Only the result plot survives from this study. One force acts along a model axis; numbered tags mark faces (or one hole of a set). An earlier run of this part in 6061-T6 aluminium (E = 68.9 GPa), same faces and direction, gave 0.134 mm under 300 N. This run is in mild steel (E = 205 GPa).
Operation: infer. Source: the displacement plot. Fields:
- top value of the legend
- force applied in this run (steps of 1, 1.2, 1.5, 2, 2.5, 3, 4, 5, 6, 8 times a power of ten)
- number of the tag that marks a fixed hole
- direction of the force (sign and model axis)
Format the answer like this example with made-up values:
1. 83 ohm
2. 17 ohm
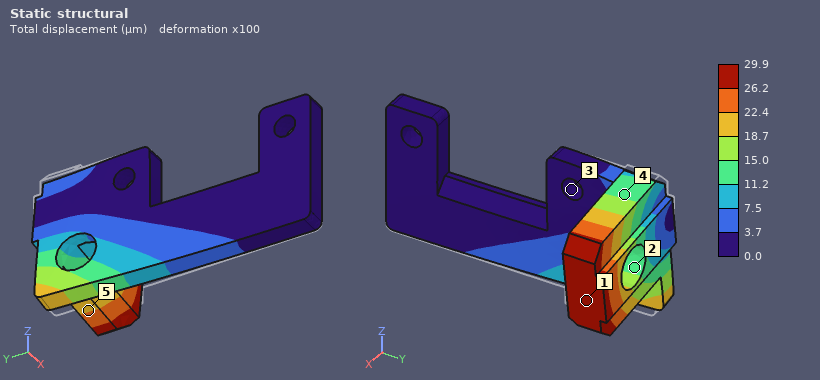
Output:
1. 29.9 µm
2. 200 N
3. 3
4. -Z
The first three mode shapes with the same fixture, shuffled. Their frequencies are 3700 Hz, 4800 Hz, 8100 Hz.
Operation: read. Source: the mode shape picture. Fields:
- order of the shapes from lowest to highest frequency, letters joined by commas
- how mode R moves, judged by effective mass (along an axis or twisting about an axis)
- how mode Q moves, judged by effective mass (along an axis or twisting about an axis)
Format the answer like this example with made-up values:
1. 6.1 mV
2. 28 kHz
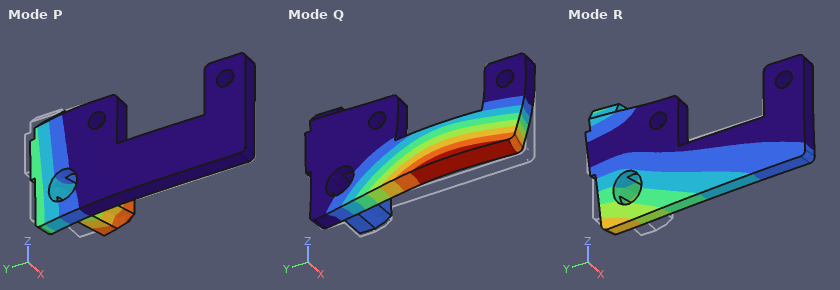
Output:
1. P, R, Q
2. along Z
3. along X
